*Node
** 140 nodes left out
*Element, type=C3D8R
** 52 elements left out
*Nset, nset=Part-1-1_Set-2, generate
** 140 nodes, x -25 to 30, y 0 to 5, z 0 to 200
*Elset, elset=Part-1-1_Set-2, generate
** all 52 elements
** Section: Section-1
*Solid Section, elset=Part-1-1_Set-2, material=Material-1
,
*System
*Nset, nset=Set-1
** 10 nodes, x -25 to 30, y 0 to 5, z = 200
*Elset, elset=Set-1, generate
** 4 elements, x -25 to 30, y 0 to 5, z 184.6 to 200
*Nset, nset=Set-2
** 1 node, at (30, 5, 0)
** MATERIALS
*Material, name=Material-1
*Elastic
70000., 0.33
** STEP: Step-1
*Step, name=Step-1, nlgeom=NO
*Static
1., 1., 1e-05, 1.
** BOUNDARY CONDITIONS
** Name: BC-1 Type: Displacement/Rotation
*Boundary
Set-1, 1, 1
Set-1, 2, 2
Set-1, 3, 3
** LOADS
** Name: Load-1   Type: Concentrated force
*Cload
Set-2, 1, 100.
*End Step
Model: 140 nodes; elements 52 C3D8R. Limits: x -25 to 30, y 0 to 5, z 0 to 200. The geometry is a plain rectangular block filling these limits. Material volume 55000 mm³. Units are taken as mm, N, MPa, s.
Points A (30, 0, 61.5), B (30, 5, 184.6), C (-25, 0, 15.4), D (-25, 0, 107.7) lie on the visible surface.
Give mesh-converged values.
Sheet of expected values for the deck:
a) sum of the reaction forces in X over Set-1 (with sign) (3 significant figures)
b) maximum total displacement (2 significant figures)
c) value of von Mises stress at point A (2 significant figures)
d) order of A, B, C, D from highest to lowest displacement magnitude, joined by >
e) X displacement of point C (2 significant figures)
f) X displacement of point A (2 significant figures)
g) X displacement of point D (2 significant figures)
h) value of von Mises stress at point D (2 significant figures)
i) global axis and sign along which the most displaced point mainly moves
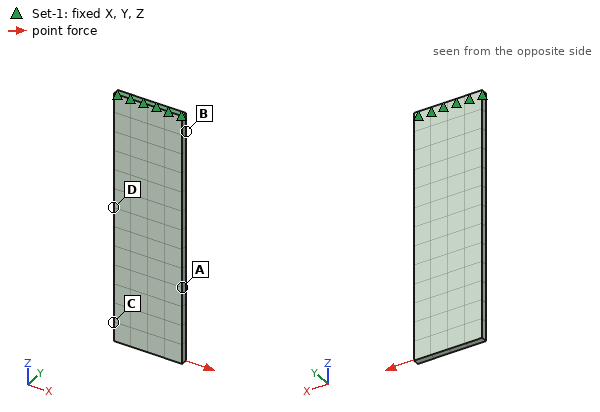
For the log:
-100 N
0.070 mm
2.5 MPa
C > A > D > B
0.049 mm
0.031 mm
0.015 mm
4.3 MPa
+X
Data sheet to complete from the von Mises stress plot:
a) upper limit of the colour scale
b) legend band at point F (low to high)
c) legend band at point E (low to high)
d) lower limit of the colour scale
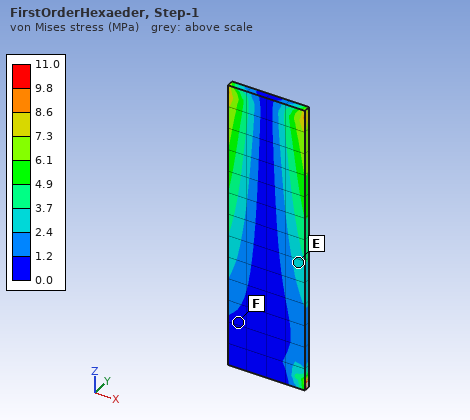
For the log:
11.0 MPa
0.0 to 1.2 MPa
2.4 to 3.7 MPa
0.0 MPa
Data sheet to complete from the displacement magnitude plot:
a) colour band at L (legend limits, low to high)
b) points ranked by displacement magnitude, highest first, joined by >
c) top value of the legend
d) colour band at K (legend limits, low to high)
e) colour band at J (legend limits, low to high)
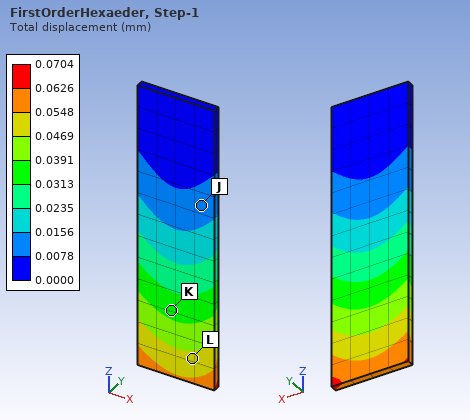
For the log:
0.0469 to 0.0548 mm
L > K > J
0.0704 mm
0.0313 to 0.0391 mm
0.0078 to 0.0156 mm
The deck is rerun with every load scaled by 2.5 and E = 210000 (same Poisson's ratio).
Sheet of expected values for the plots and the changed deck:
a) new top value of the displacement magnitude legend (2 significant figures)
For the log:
0.059 mm
